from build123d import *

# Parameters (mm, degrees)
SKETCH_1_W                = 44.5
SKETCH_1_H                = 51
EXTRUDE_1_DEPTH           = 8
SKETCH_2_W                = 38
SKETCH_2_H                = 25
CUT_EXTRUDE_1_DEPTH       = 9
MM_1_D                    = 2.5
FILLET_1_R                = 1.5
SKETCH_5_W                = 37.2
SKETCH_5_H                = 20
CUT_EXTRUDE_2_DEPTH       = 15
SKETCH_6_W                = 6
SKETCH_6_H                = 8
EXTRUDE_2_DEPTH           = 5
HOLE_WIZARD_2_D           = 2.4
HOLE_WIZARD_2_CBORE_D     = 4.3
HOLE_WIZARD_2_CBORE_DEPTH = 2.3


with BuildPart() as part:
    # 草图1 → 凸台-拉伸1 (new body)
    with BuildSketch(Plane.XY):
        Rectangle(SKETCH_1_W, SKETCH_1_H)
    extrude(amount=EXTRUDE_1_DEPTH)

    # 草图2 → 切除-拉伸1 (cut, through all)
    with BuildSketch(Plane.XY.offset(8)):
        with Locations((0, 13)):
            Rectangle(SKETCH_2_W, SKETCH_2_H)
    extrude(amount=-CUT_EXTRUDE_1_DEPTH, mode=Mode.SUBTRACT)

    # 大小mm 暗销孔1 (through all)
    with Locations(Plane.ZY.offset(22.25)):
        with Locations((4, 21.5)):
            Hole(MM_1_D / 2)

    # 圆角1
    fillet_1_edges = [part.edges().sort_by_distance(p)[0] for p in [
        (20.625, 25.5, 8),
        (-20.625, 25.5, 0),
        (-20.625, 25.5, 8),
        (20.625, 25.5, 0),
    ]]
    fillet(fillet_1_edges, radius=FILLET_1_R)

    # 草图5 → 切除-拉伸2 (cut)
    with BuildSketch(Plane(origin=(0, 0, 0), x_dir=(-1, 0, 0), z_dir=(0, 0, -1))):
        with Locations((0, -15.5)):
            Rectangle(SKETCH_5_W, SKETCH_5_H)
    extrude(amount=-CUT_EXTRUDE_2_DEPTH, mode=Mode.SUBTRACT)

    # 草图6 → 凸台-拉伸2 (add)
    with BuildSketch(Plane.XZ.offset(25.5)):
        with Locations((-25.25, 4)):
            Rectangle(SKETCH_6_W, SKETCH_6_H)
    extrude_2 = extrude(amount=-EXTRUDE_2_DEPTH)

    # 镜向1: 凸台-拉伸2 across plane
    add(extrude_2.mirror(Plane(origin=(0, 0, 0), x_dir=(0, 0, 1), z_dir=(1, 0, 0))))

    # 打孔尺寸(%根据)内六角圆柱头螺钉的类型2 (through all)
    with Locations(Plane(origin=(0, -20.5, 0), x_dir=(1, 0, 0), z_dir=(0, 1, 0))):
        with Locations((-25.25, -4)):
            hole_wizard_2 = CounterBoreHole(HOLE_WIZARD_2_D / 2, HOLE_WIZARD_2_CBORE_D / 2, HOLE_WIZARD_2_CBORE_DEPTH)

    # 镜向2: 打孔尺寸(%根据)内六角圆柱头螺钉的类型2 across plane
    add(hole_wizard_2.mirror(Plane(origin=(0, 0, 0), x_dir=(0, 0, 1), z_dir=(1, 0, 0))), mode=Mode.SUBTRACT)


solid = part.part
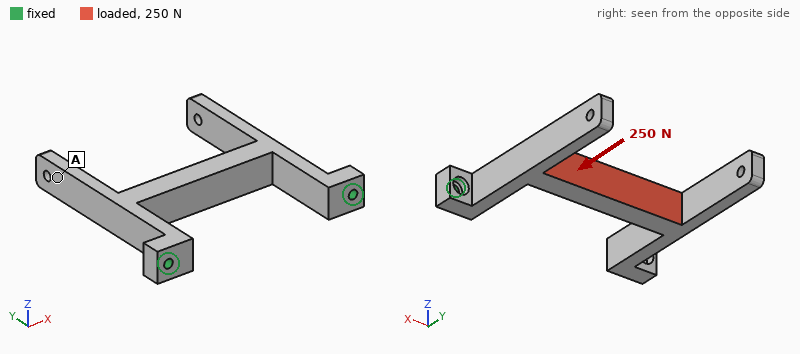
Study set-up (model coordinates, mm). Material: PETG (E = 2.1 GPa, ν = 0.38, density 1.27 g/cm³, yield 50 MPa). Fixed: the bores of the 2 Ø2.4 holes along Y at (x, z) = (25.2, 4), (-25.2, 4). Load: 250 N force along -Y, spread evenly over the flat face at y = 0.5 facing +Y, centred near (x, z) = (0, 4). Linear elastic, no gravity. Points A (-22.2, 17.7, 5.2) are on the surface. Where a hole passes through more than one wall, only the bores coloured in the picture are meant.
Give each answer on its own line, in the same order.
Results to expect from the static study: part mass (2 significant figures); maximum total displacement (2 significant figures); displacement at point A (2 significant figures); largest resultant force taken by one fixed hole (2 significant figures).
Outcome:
6.3 g
0.78 mm
0.55 mm
130 N
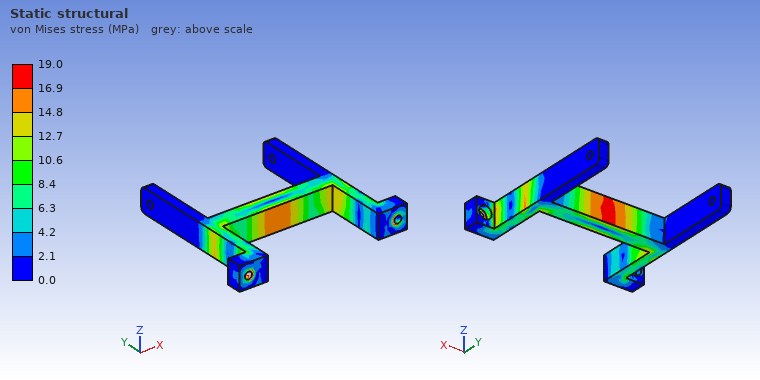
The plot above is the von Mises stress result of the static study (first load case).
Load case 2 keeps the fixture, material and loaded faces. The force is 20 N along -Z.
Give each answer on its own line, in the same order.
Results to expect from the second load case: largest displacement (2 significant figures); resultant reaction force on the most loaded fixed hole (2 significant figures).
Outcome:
0.91 mm
10 N
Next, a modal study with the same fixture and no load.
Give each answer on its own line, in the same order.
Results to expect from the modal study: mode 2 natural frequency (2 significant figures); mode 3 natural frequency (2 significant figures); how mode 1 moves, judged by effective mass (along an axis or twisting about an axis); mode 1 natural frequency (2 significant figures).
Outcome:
700 Hz
710 Hz
along Z
430 Hz
